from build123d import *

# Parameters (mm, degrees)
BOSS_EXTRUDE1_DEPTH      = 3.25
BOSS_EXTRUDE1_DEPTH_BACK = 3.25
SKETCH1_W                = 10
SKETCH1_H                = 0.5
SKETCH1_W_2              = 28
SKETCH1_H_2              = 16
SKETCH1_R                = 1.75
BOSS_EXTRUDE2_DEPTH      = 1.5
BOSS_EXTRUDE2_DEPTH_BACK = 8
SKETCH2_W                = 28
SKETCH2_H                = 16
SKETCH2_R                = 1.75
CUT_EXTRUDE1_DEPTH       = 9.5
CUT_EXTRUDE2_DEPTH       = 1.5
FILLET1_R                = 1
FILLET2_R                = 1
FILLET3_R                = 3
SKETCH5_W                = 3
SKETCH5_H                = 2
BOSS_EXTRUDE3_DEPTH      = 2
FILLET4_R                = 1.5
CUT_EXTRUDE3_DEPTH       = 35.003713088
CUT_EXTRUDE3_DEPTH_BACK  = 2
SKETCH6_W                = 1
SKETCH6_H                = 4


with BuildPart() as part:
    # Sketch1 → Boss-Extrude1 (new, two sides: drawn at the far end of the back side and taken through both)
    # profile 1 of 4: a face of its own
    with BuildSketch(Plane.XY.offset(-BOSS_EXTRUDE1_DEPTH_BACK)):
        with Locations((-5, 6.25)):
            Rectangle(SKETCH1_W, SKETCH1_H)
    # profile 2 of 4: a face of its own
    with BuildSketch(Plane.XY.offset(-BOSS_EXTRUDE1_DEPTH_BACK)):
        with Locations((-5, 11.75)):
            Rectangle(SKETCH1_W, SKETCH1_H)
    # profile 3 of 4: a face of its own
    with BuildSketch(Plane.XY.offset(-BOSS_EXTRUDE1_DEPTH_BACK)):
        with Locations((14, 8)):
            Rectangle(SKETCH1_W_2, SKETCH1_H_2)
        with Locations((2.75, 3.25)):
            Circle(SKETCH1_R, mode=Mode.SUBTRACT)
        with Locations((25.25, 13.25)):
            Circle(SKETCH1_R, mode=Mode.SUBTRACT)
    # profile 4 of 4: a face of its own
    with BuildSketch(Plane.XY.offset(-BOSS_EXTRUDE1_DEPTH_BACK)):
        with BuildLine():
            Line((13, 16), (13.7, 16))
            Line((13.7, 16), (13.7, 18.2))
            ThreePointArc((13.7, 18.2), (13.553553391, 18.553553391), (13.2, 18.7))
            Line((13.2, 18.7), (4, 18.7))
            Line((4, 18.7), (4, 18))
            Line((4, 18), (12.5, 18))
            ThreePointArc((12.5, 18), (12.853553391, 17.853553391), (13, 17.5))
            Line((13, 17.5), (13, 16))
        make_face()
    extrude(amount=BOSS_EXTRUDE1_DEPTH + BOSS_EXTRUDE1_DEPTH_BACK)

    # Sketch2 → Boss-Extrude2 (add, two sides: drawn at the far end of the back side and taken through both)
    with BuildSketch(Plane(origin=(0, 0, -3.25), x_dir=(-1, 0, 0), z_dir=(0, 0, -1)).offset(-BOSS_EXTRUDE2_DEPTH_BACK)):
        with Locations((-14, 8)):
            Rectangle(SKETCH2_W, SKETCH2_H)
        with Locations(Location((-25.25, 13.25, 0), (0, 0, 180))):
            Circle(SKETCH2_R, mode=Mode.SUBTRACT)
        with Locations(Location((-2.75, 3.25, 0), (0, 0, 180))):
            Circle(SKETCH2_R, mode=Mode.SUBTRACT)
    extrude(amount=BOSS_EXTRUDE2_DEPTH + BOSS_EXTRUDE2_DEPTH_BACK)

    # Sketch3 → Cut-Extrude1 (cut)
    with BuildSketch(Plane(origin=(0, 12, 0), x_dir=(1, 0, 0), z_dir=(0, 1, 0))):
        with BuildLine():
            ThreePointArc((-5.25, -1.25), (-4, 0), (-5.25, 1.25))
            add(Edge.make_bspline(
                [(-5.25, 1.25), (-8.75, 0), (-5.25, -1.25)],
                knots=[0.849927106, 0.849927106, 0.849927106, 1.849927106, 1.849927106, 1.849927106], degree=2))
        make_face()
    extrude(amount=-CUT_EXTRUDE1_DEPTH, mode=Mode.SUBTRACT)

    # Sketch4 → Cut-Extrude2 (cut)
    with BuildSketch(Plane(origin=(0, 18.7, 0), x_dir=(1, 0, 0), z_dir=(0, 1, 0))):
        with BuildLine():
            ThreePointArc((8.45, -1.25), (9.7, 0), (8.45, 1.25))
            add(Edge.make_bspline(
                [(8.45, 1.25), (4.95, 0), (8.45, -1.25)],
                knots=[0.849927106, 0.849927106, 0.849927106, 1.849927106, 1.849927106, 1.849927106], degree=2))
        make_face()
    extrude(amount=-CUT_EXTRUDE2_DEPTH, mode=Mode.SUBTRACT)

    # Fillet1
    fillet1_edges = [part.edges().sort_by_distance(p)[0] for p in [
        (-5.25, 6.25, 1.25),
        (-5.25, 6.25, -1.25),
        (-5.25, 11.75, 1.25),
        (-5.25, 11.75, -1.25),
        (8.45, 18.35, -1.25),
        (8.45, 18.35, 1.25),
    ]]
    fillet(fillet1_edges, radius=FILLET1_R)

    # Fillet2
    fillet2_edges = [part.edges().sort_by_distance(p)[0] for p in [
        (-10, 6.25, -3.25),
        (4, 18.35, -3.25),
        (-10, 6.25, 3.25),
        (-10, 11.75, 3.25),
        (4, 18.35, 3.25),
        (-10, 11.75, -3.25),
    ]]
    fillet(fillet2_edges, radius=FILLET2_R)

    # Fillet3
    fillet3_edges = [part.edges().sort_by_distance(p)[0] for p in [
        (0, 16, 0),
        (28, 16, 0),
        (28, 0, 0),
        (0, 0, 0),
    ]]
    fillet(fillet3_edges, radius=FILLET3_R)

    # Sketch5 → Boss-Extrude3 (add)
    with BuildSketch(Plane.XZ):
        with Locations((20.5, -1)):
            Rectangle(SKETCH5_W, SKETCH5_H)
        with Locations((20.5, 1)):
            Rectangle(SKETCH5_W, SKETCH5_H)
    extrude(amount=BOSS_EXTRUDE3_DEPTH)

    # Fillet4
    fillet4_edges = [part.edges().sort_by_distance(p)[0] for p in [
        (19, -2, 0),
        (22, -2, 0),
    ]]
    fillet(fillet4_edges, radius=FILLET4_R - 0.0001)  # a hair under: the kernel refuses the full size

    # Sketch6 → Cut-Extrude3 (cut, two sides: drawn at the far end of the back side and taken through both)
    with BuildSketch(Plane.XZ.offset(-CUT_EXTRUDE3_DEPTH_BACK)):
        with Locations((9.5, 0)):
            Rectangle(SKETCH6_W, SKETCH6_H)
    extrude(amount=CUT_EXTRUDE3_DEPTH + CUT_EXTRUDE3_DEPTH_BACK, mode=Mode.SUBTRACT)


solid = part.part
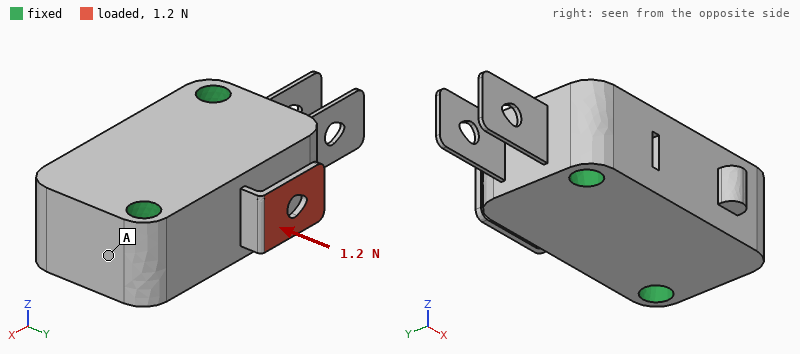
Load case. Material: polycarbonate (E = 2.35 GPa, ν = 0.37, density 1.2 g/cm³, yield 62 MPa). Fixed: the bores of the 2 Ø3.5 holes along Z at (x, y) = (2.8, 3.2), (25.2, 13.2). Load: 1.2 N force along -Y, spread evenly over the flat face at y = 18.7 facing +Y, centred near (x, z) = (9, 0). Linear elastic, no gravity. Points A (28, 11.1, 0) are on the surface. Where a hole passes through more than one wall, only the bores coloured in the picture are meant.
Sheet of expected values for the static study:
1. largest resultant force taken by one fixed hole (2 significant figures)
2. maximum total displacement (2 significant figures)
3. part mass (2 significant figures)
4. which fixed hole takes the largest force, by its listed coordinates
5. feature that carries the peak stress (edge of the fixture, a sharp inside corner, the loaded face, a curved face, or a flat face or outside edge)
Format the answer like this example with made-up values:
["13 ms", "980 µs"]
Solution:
["0.94 N", "0.50 mm", "4.9 g", "(2.8, 3.2)", "a curved face"]
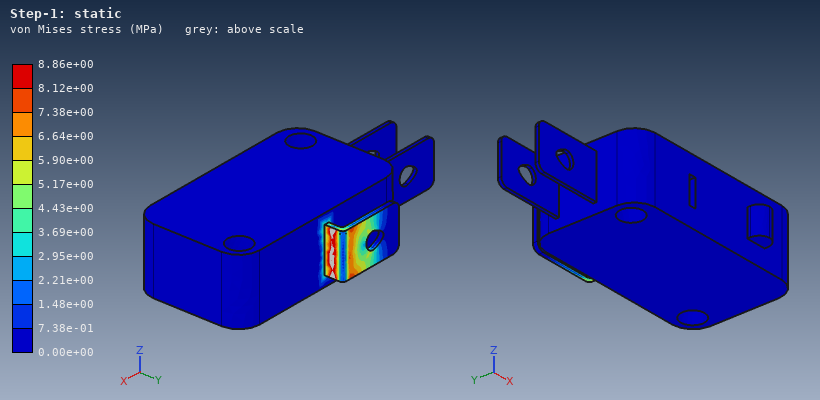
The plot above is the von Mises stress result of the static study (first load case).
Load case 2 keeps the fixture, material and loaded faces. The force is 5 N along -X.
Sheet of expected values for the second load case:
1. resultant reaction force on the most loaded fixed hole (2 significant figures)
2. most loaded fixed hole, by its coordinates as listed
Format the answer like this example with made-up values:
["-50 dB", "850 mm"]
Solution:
["3.8 N", "(25.2, 13.2)"]
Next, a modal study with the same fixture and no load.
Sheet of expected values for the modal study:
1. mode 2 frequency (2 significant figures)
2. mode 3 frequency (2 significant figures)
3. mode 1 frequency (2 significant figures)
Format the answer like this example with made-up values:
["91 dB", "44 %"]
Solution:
["1200 Hz", "1400 Hz", "1100 Hz"]
